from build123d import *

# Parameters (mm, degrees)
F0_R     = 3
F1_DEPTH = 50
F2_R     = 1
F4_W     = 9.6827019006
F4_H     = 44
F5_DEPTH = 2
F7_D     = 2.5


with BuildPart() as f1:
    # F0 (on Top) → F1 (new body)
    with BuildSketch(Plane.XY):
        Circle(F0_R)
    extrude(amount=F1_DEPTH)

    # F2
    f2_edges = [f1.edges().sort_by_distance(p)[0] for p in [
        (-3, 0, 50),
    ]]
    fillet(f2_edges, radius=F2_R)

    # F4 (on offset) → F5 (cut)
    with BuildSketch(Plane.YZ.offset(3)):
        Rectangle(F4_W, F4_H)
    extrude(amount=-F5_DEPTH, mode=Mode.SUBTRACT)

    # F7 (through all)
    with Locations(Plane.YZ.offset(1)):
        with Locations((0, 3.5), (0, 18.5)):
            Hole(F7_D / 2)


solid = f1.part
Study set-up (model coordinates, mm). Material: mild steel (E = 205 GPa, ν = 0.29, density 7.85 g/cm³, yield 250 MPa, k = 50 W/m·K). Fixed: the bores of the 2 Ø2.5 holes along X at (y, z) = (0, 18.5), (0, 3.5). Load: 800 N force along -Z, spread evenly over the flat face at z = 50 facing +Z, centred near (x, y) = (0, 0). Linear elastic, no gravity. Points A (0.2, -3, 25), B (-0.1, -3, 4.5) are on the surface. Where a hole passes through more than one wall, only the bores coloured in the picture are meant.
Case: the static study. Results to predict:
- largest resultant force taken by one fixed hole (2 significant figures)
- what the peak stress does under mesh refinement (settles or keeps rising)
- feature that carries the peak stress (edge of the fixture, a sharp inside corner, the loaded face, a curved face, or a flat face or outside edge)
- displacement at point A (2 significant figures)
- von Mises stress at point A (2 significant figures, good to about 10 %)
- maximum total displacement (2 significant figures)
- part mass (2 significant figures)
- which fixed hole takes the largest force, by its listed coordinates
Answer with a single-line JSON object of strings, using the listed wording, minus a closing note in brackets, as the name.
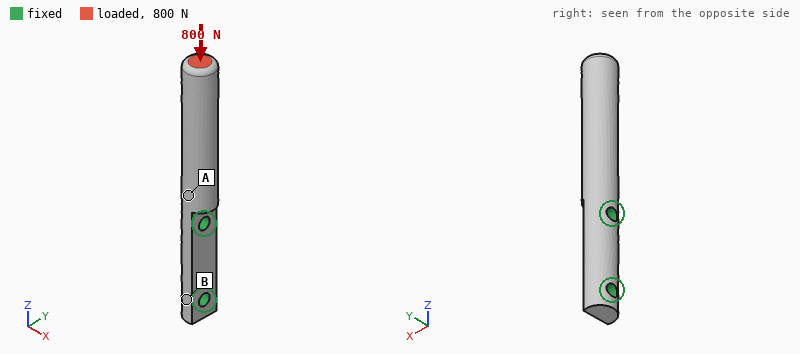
{"largest resultant force taken by one fixed hole": "780 N", "what the peak stress does under mesh refinement": "keeps rising", "feature that carries the peak stress": "edge of the fixture", "displacement at point A": "2.7 µm", "von Mises stress at point A": "36 MPa", "maximum total displacement": "17 µm", "part mass": "9.3 g", "which fixed hole takes the largest force, by its listed coordinates": "(0, 18.5)"}
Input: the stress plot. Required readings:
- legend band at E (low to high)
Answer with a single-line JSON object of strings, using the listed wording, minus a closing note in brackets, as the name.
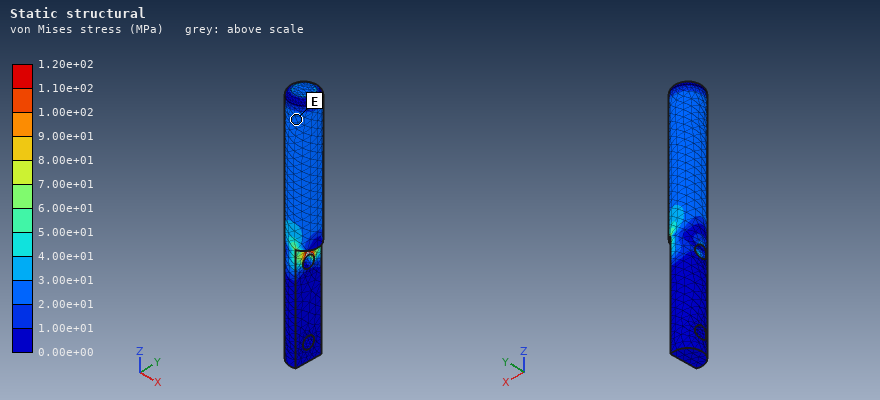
{"legend band at E": "2.00e+01 to 3.00e+01 MPa"}
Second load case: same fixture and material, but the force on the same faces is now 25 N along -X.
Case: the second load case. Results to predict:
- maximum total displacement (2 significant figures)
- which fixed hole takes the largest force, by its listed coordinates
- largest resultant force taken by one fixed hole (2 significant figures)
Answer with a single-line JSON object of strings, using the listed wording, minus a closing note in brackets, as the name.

{"maximum total displacement": "31 µm", "which fixed hole takes the largest force, by its listed coordinates": "(0, 18.5)", "largest resultant force taken by one fixed hole": "27 N"}
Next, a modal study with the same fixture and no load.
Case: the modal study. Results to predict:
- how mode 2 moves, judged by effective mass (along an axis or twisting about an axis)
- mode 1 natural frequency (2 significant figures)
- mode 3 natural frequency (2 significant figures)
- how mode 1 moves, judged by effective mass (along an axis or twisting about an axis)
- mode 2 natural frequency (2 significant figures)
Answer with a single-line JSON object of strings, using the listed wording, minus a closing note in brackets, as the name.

{"how mode 2 moves, judged by effective mass": "along Y", "mode 1 natural frequency": "3400 Hz", "mode 3 natural frequency": "22 kHz", "how mode 1 moves, judged by effective mass": "along X", "mode 2 natural frequency": "3800 Hz"}
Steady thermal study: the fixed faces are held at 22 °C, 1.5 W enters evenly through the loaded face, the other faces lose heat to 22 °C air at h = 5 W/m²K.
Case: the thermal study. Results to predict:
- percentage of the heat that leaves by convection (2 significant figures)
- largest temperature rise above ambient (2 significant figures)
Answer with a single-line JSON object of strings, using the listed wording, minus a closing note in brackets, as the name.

{"percentage of the heat that leaves by convection": "3.5 %", "largest temperature rise above ambient": "35 K"}
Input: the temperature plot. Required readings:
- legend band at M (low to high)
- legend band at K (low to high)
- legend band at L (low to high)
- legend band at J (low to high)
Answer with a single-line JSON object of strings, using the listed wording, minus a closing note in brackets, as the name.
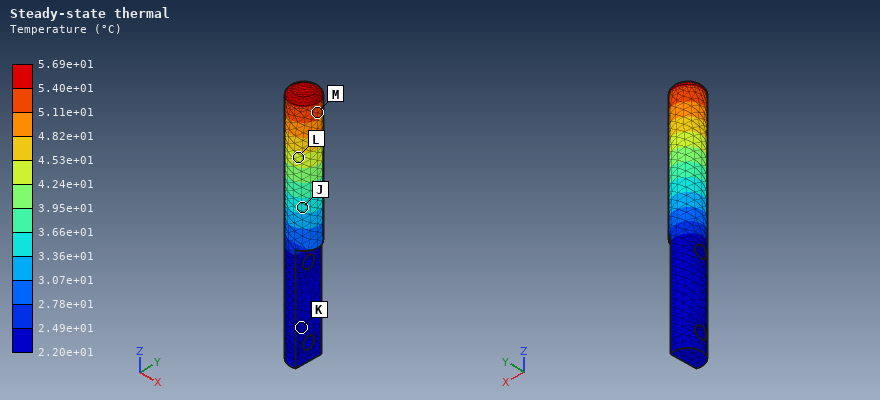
{"legend band at M": "5.11e+01 to 5.40e+01 °C", "legend band at K": "2.20e+01 to 2.49e+01 °C", "legend band at L": "4.24e+01 to 4.53e+01 °C", "legend band at J": "3.36e+01 to 3.66e+01 °C"}
